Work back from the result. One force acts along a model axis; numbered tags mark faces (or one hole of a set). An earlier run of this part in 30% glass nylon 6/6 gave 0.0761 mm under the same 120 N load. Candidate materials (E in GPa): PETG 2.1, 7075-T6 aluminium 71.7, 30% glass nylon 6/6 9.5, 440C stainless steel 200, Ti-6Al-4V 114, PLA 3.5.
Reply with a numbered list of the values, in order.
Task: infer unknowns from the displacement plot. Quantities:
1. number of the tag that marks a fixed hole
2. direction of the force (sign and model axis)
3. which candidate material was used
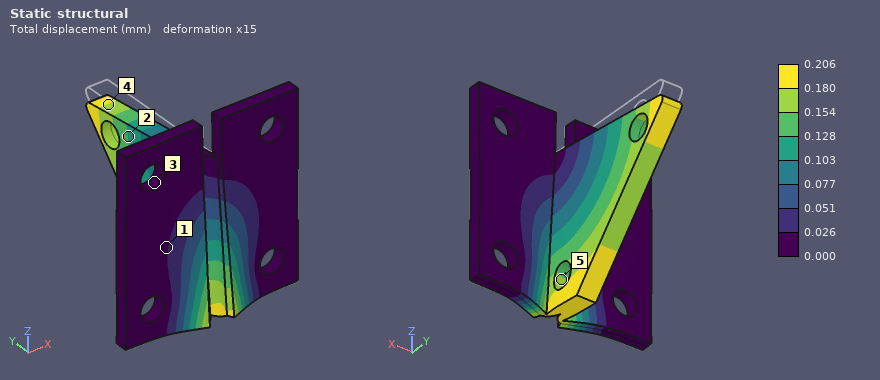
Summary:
1. 3
2. -Y
3. PLA
